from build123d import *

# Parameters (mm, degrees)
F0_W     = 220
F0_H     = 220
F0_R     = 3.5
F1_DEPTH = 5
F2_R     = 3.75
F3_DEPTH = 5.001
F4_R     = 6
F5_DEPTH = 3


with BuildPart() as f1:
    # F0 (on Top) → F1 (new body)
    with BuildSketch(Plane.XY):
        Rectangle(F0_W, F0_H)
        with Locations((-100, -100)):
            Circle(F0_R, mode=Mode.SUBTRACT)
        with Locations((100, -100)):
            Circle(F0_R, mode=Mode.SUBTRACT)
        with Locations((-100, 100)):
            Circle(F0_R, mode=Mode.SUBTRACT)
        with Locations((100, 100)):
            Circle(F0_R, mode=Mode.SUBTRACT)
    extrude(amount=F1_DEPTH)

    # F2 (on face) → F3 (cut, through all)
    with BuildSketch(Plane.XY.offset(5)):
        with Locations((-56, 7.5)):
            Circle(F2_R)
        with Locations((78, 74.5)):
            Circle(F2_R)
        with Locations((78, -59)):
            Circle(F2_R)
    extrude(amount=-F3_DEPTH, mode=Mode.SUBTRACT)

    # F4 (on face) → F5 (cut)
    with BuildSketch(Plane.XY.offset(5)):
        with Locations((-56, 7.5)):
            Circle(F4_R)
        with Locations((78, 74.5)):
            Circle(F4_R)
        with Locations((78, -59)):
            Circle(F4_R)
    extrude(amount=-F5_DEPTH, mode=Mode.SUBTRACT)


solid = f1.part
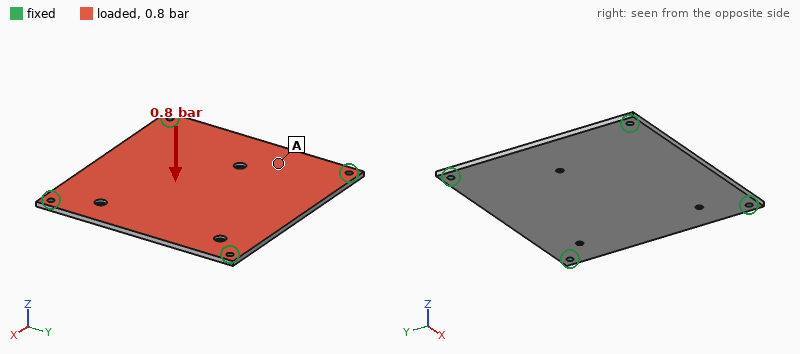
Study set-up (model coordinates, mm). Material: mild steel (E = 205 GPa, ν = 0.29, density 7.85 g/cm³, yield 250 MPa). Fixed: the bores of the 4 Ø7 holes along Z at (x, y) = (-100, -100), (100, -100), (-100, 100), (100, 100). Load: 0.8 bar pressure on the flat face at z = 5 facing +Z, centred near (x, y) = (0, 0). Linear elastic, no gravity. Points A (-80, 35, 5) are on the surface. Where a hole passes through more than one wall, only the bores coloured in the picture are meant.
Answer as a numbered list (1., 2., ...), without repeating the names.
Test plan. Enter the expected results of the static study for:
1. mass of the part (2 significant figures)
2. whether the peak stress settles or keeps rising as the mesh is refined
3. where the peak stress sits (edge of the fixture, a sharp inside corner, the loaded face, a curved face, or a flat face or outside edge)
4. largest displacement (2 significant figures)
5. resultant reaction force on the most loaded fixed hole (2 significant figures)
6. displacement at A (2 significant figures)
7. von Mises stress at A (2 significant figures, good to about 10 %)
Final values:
1. 1.9 kg
2. keeps rising
3. edge of the fixture
4. 0.49 mm
5. 960 N
6. 0.28 mm
7. 34 MPa
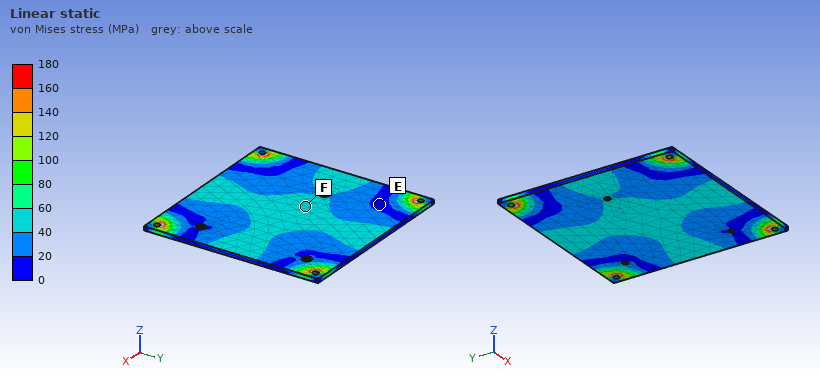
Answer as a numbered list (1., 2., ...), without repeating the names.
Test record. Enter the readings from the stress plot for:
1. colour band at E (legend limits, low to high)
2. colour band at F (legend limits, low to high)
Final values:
1. 0 to 20 MPa
2. 40 to 60 MPa
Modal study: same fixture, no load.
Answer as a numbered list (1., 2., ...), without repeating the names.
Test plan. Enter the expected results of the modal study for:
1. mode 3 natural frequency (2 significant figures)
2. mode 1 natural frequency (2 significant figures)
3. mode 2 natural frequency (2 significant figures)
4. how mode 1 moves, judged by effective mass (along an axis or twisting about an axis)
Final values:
1. 710 Hz
2. 390 Hz
3. 710 Hz
4. along Z
